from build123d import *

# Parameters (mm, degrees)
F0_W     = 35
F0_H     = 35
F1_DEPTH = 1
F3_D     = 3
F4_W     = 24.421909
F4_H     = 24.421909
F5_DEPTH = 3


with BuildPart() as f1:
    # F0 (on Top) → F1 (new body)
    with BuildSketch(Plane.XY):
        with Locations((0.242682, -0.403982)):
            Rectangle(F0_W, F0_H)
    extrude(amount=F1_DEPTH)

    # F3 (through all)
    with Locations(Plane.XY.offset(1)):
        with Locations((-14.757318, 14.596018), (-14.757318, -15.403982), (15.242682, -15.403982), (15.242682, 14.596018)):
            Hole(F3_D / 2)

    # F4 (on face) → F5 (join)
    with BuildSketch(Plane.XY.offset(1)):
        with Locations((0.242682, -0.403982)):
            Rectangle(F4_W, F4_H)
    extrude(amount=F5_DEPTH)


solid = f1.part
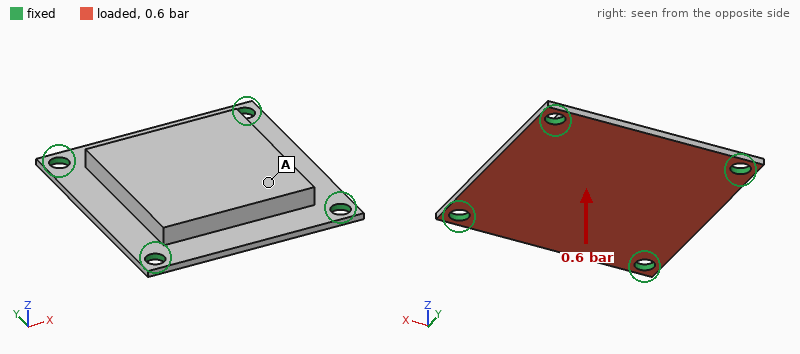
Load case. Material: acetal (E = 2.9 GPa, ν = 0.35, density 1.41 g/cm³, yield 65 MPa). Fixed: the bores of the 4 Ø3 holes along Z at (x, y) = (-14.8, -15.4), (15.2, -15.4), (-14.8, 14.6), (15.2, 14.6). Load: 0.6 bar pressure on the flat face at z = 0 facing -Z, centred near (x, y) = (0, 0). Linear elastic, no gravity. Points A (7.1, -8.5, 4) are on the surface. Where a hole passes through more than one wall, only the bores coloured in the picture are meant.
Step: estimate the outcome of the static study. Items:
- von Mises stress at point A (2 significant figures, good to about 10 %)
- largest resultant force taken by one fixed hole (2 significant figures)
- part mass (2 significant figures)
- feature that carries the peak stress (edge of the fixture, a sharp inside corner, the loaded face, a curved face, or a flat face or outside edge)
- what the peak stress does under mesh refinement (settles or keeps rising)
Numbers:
2.6 MPa
25 N
4.2 g
edge of the fixture
keeps rising
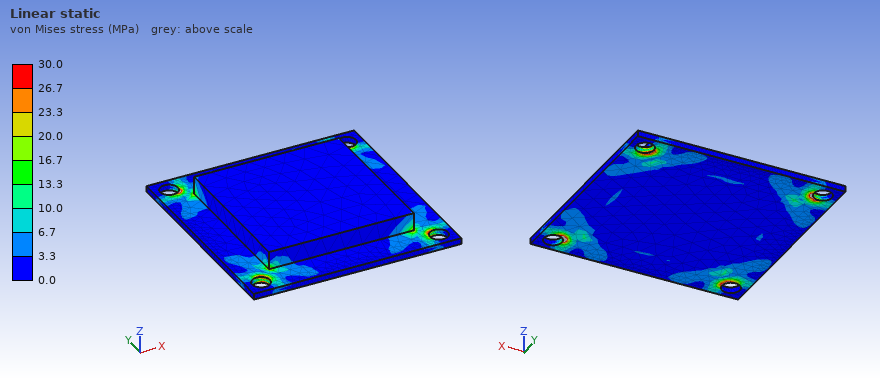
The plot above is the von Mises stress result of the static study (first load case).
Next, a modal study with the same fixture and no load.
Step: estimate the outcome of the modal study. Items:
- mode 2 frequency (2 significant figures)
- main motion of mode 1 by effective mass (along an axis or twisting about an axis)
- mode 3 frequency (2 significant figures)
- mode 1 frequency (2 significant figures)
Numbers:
3500 Hz
along Z
3500 Hz
2100 Hz
